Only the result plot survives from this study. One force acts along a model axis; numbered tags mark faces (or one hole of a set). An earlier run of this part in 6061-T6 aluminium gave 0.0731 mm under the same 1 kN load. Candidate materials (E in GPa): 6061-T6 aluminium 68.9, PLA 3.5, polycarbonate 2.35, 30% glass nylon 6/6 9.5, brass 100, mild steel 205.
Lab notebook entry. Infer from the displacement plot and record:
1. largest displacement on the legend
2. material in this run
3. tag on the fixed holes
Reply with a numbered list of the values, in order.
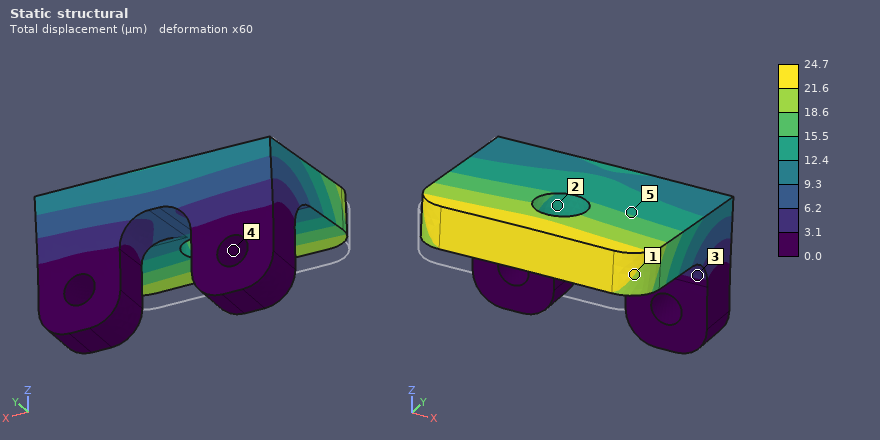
1. 24.7 µm
2. mild steel
3. 4
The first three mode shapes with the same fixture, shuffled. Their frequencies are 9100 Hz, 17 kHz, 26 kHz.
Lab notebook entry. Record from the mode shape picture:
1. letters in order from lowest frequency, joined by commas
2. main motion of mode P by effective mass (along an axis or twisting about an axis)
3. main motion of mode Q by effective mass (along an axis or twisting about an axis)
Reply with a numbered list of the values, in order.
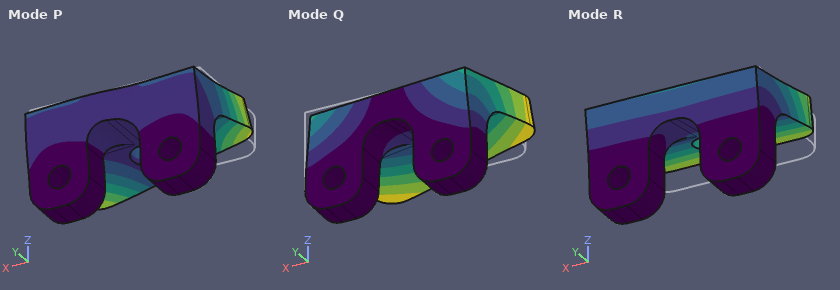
1. R, Q, P
2. along X
3. along X
